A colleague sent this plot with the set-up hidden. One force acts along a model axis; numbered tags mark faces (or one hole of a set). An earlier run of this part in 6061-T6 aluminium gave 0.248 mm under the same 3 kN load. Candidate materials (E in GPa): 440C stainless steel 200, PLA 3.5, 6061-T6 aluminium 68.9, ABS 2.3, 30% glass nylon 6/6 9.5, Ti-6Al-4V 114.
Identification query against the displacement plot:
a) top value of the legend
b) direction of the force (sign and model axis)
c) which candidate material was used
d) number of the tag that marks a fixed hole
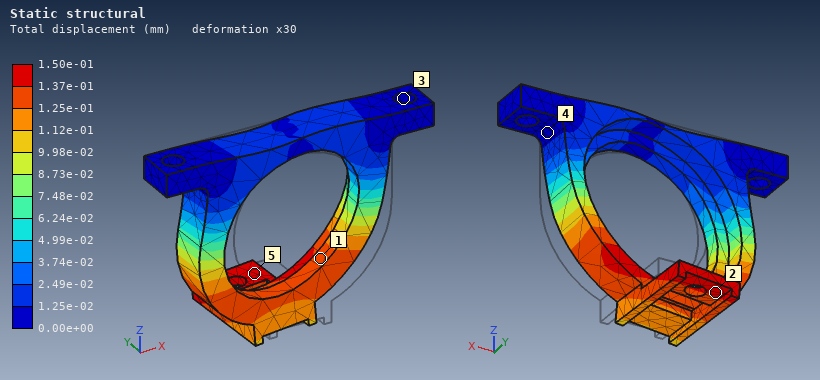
1.50e-01 mm
-X
Ti-6Al-4V
3
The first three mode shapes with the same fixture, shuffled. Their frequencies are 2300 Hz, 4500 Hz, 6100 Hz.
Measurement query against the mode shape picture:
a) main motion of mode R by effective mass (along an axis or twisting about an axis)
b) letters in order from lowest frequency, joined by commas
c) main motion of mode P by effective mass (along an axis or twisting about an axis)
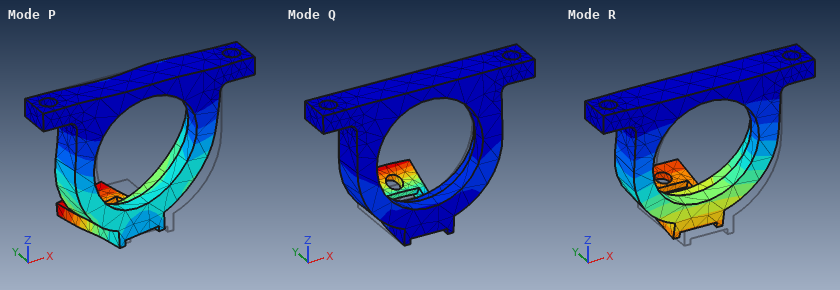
along Y
R, P, Q
along X
